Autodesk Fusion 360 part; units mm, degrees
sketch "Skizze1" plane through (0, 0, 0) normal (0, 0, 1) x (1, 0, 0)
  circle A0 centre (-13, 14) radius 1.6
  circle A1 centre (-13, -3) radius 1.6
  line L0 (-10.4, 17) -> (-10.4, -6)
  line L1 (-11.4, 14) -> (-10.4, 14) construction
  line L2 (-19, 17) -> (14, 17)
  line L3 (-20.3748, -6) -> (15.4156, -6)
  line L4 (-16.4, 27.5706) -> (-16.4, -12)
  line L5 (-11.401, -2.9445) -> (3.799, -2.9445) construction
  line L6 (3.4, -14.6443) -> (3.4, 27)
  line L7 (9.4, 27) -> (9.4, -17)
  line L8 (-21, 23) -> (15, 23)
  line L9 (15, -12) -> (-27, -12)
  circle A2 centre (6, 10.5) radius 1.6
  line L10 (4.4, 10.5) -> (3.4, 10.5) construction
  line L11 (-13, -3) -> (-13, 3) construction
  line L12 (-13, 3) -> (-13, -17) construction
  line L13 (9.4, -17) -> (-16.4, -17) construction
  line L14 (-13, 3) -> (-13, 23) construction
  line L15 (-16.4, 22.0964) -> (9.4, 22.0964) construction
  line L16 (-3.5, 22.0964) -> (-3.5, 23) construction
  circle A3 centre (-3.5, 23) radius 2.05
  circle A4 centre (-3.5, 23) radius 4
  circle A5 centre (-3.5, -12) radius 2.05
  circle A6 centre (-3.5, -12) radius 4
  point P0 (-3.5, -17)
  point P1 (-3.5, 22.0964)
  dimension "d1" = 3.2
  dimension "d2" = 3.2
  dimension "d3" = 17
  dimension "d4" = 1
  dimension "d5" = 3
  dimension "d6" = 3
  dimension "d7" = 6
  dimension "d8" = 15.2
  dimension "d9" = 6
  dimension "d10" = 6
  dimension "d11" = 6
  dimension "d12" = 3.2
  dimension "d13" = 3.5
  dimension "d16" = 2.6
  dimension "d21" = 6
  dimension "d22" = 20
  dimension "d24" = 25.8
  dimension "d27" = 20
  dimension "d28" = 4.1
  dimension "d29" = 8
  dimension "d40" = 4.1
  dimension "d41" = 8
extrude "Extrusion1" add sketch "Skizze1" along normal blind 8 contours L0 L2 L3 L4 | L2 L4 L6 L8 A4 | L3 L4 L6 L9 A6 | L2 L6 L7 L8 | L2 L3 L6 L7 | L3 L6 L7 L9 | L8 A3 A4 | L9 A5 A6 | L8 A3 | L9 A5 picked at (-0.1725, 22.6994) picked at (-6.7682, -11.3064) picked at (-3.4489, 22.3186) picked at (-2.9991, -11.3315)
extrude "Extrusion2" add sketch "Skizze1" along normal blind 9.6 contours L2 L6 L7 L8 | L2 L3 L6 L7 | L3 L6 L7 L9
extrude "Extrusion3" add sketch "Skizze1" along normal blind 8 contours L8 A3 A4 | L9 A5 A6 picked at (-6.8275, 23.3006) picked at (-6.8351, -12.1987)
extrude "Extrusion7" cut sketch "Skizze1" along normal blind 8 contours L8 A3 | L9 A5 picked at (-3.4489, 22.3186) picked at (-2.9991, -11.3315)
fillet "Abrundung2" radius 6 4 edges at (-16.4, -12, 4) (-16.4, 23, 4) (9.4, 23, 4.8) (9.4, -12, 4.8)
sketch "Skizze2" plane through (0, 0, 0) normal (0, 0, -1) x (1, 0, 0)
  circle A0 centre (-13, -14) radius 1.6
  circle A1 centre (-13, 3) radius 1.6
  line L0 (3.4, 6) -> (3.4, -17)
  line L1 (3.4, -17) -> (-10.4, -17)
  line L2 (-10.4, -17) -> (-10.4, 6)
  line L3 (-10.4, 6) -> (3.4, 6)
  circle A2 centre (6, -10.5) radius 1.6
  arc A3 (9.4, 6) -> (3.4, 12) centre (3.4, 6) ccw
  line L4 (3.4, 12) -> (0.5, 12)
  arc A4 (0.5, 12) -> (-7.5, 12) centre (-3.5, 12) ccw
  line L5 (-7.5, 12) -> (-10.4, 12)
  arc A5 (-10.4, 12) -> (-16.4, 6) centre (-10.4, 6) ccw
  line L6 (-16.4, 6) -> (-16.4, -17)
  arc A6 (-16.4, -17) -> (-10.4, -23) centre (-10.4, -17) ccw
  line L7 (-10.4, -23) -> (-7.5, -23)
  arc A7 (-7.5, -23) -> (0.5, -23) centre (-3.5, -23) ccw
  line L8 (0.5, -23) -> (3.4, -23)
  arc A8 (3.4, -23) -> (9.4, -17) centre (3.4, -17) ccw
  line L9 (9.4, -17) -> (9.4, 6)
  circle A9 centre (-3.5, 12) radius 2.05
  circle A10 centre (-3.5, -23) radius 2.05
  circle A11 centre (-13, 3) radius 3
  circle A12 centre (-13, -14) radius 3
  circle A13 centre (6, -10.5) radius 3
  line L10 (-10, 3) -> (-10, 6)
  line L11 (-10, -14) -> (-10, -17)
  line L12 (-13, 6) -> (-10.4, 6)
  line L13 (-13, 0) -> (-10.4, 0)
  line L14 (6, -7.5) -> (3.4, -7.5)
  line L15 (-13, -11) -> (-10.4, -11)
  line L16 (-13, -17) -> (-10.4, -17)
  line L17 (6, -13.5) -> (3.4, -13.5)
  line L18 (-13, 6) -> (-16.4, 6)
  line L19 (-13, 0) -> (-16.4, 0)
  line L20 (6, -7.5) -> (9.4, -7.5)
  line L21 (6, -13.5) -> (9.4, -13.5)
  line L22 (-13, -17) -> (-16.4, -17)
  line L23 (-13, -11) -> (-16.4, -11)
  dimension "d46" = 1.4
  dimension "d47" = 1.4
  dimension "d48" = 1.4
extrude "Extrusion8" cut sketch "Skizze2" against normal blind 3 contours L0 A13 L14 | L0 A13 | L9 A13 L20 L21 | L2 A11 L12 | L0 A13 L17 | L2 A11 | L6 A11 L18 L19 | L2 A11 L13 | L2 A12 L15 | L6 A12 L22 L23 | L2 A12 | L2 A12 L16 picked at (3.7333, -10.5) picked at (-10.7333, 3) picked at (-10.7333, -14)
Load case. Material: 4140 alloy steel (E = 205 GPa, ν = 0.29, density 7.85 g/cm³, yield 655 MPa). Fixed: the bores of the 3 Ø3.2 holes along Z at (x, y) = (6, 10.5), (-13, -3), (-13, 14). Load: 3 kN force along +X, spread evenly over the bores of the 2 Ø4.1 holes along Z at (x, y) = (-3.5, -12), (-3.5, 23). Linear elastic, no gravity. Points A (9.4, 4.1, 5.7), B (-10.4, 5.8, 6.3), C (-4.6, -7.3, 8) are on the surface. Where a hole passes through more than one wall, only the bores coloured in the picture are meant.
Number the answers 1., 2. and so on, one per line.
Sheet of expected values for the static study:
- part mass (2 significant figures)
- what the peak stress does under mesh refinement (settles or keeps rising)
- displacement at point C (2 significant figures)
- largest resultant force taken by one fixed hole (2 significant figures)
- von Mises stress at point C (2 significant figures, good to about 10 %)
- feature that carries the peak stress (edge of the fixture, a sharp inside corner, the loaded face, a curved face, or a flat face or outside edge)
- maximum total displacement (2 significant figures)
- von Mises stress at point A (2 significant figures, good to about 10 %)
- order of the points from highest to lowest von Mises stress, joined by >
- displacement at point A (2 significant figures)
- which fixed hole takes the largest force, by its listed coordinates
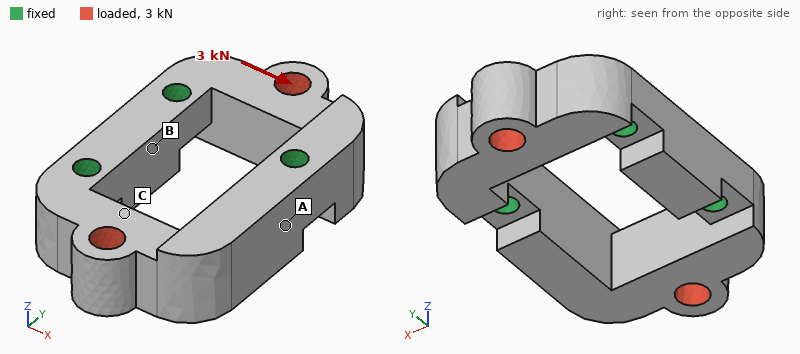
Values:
1. 35 g
2. keeps rising
3. 4.5 µm
4. 1.4 kN
5. 44 MPa
6. edge of the fixture
7. 7.0 µm
8. 24 MPa
9. C > A > B
10. 1.8 µm
11. (-13, -3)
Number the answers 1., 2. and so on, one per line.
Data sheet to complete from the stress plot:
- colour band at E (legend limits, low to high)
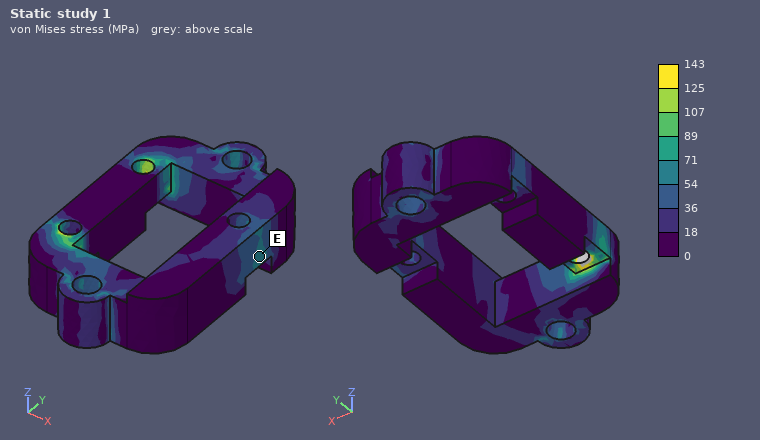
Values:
1. 54 to 71 MPa
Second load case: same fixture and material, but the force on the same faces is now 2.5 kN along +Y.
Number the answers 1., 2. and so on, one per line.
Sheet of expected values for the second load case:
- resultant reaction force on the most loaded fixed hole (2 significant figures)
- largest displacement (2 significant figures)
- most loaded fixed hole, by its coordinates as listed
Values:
1. 1.3 kN
2. 6.8 µm
3. (6, 10.5)
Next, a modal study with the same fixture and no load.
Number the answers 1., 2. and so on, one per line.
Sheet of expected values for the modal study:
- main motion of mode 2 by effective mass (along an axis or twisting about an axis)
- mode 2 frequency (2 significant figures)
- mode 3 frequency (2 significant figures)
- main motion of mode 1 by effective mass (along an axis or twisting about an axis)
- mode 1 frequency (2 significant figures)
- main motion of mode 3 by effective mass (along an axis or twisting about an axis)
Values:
1. along Z
2. 20 kHz
3. 24 kHz
4. along Z
5. 11 kHz
6. along X
